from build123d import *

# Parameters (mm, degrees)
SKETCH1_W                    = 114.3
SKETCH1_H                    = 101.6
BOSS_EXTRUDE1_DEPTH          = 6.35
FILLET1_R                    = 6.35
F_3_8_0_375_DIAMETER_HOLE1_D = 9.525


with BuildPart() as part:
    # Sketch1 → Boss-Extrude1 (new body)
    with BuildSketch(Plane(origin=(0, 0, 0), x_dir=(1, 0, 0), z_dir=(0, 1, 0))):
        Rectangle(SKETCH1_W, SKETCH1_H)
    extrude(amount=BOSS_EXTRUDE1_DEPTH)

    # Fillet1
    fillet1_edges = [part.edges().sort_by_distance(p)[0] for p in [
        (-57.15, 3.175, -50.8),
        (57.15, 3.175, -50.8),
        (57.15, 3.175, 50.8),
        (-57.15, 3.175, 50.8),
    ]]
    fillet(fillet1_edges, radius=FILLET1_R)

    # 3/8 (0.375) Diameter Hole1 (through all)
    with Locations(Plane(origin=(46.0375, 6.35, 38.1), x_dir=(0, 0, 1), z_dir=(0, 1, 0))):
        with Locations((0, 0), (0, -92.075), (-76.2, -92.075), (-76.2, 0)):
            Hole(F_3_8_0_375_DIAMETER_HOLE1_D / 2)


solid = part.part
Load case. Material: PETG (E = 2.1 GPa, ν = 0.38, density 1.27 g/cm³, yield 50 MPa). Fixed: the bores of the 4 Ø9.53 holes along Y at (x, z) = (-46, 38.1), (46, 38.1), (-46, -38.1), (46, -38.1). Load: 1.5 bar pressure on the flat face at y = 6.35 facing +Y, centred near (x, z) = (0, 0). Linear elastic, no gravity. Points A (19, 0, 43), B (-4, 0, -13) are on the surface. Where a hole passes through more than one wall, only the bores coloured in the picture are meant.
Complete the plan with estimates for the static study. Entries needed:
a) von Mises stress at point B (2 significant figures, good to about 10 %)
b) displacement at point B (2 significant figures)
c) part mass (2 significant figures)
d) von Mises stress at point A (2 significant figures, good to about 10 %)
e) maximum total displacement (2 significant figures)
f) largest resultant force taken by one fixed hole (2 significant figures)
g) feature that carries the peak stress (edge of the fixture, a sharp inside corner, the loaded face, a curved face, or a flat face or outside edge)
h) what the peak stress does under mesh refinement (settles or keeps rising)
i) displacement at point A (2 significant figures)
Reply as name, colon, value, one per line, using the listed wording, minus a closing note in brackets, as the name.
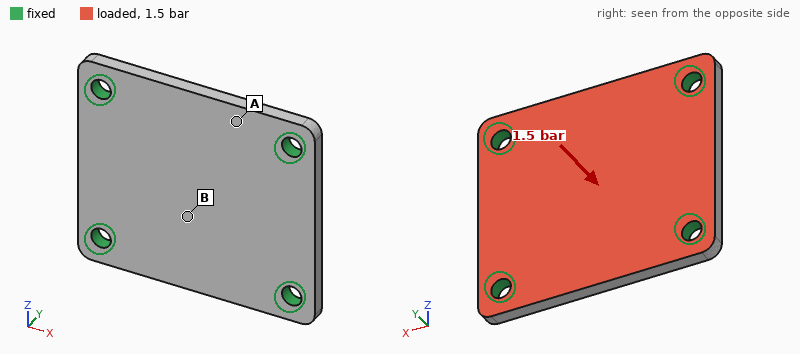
von Mises stress at point B: 7.5 MPa
displacement at point B: 0.86 mm
part mass: 91 g
von Mises stress at point A: 3.5 MPa
maximum total displacement: 0.91 mm
largest resultant force taken by one fixed hole: 420 N
feature that carries the peak stress: edge of the fixture
what the peak stress does under mesh refinement: keeps rising
displacement at point A: 0.41 mm
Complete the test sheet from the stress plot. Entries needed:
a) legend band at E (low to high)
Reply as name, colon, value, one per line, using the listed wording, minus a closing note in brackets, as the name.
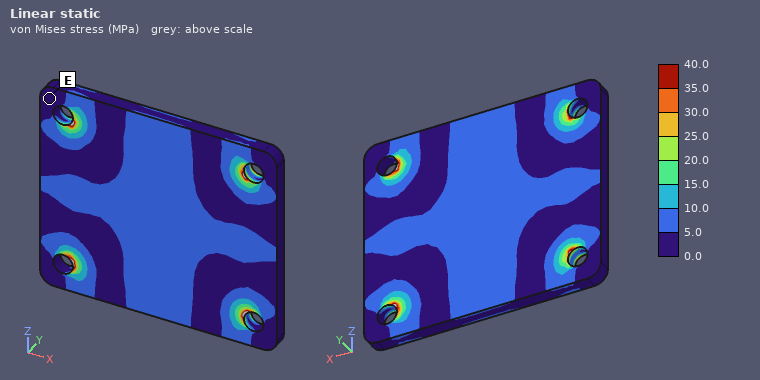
legend band at E: 0.0 to 5.0 MPa
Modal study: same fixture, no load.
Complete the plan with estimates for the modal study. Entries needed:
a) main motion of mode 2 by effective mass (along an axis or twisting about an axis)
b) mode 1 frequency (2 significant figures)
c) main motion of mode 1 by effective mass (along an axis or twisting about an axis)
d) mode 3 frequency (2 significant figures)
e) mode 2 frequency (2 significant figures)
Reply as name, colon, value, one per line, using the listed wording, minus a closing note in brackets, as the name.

main motion of mode 2 by effective mass: twisting about X
mode 1 frequency: 870 Hz
main motion of mode 1 by effective mass: along Y
mode 3 frequency: 1500 Hz
mode 2 frequency: 1200 Hz
